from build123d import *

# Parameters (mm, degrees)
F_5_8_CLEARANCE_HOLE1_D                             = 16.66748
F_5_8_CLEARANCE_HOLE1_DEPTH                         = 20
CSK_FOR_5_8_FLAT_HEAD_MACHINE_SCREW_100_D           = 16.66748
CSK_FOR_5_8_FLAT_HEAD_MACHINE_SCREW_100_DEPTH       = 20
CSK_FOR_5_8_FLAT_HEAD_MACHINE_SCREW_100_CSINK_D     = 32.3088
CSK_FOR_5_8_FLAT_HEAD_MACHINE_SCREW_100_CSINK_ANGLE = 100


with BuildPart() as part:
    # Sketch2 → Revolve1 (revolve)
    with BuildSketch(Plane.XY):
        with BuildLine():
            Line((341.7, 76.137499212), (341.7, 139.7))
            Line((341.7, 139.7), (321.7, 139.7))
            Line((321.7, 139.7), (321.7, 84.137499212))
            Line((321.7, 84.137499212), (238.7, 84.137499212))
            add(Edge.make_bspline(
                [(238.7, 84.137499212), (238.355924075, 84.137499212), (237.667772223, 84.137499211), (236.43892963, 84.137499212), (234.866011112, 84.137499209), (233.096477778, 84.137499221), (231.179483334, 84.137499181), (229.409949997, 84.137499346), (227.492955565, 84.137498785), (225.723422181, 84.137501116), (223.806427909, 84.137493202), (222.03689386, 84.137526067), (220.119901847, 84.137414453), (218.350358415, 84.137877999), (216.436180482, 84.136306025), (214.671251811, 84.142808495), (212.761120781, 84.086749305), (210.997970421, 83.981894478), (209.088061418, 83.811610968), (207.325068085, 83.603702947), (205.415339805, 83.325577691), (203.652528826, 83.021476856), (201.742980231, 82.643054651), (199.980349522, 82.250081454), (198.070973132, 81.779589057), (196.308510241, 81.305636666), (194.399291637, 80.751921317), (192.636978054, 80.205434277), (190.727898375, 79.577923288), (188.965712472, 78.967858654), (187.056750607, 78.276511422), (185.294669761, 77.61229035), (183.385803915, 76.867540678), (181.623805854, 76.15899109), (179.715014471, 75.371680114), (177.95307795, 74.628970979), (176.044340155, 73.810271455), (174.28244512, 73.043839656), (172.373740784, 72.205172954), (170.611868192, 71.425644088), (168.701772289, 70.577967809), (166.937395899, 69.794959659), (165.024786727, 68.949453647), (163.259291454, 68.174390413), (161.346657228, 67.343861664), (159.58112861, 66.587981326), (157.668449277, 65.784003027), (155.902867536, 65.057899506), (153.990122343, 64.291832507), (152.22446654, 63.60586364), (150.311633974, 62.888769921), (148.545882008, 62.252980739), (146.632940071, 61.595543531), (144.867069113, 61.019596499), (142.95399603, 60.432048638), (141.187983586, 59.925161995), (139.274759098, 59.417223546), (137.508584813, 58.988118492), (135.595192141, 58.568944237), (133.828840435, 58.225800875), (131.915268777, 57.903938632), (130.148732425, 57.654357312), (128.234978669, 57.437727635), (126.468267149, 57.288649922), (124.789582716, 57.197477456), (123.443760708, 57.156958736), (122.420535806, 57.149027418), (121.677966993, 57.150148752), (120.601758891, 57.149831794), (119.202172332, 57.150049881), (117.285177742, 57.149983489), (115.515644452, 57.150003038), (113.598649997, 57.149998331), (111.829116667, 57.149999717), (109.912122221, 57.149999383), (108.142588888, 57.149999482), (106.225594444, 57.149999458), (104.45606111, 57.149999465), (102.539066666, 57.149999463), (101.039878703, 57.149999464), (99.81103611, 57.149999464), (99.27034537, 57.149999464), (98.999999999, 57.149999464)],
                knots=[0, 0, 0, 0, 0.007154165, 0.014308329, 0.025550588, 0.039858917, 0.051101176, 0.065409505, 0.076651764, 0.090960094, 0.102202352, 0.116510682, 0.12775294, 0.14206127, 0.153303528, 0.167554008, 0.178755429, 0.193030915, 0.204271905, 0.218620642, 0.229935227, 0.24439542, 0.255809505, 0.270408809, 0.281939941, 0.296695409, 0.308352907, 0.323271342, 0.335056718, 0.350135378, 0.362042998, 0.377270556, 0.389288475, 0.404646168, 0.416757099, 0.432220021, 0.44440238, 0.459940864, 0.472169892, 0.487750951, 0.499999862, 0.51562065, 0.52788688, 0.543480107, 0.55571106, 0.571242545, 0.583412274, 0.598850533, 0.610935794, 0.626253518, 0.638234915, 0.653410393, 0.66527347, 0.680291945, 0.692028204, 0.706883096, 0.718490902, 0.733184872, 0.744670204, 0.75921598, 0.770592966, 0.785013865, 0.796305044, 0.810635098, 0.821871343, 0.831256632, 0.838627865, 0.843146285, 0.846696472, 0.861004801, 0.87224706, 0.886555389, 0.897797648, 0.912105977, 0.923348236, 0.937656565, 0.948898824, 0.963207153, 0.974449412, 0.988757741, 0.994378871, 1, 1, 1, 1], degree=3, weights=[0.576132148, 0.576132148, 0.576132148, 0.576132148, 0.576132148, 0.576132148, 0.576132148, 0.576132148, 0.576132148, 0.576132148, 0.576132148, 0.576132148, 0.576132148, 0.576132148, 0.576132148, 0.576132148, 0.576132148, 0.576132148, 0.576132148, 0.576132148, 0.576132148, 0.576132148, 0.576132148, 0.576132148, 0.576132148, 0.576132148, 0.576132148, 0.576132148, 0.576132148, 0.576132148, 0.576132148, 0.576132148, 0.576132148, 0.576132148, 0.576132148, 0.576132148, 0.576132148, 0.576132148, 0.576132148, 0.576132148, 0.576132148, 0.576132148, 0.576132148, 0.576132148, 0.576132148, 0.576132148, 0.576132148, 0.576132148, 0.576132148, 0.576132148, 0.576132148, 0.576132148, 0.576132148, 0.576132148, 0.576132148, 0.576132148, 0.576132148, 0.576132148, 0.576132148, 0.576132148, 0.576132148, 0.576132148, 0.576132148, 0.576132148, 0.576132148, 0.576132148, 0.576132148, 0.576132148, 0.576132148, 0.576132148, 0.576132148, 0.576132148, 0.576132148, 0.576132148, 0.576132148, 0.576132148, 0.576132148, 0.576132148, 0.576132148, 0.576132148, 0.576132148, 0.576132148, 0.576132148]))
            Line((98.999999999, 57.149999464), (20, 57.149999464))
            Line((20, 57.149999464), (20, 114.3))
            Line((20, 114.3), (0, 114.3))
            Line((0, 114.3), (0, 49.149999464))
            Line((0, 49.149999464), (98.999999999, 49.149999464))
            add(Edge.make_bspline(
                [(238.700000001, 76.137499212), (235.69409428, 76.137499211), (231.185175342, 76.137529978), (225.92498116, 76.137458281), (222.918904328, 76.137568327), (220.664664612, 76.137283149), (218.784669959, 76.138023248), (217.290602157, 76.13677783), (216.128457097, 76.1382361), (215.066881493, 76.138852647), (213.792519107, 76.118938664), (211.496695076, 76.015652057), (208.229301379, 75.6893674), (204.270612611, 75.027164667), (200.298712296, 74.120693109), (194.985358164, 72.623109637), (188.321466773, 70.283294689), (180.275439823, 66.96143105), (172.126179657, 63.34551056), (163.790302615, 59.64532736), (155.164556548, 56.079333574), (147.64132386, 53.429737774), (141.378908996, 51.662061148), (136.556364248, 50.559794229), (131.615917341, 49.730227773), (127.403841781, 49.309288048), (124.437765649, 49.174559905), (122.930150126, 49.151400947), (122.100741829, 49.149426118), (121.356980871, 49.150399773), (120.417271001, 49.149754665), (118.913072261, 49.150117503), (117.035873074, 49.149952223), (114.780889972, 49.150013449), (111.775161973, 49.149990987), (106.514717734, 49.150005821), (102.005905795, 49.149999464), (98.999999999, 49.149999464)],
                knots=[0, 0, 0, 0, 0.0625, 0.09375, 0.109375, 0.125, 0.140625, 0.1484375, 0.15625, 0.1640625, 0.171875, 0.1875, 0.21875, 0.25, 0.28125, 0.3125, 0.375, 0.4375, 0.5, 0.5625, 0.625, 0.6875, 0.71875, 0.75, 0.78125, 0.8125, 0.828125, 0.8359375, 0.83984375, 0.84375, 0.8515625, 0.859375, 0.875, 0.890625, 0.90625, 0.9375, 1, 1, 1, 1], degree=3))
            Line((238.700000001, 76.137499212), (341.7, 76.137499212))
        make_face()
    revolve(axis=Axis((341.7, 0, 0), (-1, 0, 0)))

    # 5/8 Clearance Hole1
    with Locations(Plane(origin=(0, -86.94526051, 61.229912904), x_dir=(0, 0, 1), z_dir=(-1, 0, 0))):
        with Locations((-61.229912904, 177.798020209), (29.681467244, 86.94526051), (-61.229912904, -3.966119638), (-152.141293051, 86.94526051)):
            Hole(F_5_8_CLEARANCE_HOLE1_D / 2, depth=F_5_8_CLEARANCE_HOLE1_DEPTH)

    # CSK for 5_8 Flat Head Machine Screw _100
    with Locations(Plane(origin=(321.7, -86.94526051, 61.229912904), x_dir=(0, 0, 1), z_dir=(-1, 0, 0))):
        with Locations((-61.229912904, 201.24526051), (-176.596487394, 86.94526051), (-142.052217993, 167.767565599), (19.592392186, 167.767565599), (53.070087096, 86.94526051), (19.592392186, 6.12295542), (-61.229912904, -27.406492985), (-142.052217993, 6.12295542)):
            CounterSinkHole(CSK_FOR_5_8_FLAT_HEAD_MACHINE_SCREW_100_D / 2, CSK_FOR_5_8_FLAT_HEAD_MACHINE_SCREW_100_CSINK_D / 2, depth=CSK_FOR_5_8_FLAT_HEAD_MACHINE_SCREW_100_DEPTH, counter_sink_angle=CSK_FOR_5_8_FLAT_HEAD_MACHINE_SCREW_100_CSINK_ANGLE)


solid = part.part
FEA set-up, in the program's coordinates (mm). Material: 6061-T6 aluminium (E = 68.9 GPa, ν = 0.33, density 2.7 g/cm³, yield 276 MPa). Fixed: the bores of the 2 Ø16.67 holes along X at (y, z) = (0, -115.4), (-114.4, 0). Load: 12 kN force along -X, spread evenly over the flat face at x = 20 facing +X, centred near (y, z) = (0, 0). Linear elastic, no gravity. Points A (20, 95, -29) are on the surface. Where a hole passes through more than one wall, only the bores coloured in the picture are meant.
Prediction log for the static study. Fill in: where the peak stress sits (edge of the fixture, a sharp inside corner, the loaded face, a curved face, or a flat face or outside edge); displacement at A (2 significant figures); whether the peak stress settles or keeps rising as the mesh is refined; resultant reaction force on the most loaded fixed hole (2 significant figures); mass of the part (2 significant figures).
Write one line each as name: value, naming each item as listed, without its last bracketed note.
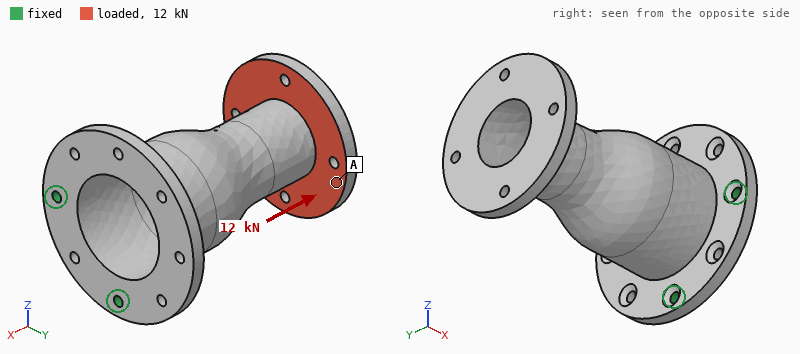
where the peak stress sits: edge of the fixture
displacement at A: 1.7 mm
whether the peak stress settles or keeps rising as the mesh is refined: keeps rising
resultant reaction force on the most loaded fixed hole: 6.0 kN
mass of the part: 6.7 kg
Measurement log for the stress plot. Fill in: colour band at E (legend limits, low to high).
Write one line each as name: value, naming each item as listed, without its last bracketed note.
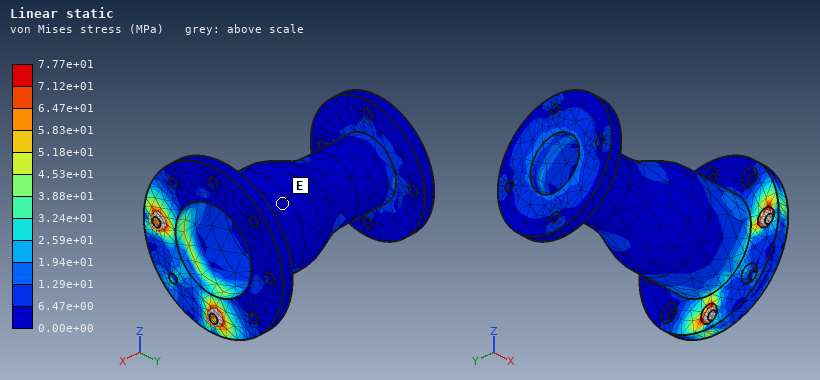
colour band at E: 0.00e+00 to 6.47e+00 MPa
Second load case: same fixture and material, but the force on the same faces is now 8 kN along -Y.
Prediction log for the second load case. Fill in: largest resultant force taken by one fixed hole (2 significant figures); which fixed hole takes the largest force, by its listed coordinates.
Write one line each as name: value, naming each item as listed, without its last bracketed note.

largest resultant force taken by one fixed hole: 15 kN
which fixed hole takes the largest force, by its listed coordinates: (-114.4, 0)
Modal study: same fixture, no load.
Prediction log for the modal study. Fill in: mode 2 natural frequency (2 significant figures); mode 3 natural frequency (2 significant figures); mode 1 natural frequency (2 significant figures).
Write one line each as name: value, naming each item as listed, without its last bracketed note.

mode 2 natural frequency: 320 Hz
mode 3 natural frequency: 930 Hz
mode 1 natural frequency: 110 Hz
